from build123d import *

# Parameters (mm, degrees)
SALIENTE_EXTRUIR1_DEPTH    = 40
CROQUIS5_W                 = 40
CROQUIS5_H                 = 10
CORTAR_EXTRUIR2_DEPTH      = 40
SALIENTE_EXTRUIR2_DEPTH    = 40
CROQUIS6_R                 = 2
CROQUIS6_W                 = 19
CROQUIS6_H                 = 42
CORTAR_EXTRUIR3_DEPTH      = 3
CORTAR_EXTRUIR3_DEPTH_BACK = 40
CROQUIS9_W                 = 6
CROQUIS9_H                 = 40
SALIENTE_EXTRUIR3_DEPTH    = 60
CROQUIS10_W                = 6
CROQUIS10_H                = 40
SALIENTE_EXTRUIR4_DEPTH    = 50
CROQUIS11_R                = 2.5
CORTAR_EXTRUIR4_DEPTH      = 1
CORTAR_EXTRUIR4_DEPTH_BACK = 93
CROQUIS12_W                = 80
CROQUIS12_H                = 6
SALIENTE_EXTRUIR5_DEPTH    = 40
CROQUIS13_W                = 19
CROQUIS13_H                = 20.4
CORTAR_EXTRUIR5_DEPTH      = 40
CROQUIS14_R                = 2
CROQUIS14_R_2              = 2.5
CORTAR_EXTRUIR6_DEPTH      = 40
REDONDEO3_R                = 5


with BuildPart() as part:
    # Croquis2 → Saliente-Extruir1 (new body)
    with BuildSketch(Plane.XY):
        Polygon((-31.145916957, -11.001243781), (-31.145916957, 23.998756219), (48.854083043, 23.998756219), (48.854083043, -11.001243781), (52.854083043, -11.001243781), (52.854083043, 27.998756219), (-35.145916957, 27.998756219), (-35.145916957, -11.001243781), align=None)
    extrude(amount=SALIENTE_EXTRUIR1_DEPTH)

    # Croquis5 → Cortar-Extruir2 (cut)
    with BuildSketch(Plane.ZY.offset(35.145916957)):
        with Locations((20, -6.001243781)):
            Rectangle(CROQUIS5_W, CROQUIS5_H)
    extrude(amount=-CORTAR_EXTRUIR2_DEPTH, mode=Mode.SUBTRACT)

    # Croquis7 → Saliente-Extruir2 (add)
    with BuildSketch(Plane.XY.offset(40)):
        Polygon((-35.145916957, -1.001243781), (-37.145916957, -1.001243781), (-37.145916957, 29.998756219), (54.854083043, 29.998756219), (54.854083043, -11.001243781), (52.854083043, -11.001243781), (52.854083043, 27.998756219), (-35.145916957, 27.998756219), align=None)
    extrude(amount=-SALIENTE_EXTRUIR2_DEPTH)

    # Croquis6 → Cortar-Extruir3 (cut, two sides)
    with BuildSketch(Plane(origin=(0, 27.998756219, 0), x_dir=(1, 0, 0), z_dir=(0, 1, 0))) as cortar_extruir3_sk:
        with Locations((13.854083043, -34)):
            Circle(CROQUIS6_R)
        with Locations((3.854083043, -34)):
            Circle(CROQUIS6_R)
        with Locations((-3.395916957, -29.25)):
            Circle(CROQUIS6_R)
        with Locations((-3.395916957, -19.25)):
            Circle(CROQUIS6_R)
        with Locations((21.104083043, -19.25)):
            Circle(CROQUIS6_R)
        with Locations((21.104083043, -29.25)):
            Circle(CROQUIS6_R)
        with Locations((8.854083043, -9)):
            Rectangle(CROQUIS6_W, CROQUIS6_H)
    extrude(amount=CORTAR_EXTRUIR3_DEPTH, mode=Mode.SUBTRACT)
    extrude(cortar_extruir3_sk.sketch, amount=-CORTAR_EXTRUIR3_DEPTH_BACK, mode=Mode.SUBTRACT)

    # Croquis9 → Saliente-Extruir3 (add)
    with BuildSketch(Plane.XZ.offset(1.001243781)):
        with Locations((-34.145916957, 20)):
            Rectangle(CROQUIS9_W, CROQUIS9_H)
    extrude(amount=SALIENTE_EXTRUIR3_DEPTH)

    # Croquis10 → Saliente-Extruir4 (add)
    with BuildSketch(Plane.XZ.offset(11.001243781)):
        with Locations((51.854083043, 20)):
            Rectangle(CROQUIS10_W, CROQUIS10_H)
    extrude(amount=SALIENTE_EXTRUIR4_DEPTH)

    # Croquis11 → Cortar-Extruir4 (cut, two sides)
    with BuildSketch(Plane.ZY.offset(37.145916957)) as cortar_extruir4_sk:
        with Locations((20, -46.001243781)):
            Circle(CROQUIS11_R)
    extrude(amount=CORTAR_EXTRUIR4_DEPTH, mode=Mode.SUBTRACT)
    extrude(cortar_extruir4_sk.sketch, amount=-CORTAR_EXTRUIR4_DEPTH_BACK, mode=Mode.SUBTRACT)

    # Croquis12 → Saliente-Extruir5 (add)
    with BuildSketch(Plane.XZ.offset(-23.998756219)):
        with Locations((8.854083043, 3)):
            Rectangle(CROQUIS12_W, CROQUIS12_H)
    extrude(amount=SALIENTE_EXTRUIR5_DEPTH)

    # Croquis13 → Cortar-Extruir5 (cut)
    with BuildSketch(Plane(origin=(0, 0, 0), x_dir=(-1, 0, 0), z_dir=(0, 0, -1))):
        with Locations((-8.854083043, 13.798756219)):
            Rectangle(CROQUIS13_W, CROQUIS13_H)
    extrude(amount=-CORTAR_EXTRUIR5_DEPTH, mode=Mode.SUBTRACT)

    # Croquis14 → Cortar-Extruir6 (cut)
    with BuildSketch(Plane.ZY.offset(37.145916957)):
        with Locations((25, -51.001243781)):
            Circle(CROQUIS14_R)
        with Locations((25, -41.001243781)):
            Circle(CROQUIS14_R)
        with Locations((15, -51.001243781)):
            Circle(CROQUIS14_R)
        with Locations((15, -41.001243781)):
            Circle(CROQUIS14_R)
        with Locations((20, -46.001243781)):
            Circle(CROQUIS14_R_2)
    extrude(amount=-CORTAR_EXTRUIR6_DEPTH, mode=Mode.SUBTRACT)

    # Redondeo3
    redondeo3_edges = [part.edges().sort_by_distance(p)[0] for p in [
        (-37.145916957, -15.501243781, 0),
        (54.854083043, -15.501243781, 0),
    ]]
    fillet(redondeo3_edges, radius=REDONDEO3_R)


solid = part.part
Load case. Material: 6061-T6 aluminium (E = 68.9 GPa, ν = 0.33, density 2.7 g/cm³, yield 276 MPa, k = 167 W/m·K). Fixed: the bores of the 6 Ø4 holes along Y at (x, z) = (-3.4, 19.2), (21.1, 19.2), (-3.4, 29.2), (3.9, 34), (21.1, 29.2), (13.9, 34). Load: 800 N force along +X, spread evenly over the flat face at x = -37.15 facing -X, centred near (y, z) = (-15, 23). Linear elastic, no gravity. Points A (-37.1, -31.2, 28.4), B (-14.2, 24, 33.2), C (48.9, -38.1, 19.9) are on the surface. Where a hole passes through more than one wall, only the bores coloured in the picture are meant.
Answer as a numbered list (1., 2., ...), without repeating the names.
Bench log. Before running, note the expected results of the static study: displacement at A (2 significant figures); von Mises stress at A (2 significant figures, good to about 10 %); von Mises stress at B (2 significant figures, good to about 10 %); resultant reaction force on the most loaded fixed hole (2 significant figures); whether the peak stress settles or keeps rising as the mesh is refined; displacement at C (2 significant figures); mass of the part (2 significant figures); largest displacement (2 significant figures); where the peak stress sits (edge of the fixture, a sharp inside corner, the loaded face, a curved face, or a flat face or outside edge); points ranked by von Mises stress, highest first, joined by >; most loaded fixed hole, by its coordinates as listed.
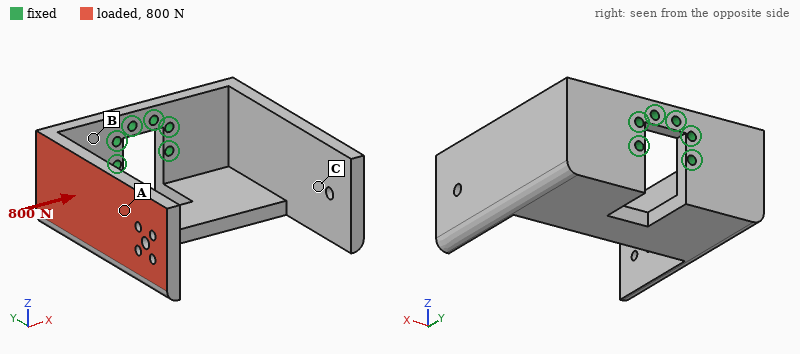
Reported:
1. 0.38 mm
2. 18 MPa
3. 38 MPa
4. 1.1 kN
5. keeps rising
6. 0.20 mm
7. 200 g
8. 0.71 mm
9. edge of the fixture
10. B > A > C
11. (21.1, 19.2)
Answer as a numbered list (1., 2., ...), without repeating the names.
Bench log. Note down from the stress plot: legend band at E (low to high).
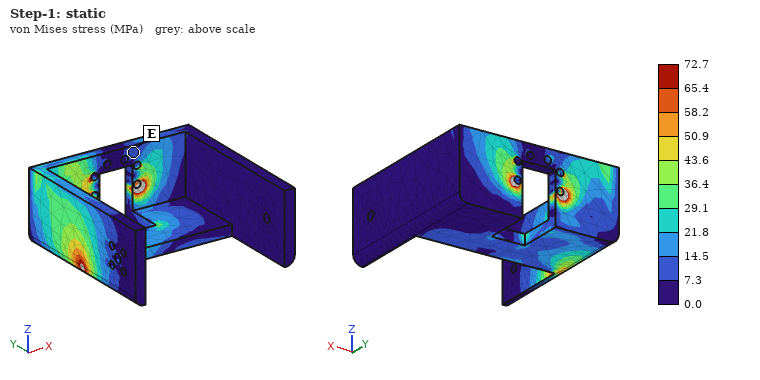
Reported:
1. 7.3 to 14.5 MPa
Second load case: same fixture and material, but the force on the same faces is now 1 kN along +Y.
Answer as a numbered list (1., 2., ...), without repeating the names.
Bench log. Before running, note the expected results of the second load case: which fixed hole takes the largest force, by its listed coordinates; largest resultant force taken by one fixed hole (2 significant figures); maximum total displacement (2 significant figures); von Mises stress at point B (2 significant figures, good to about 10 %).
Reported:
1. (-3.4, 19.2)
2. 1.3 kN
3. 0.30 mm
4. 40 MPa
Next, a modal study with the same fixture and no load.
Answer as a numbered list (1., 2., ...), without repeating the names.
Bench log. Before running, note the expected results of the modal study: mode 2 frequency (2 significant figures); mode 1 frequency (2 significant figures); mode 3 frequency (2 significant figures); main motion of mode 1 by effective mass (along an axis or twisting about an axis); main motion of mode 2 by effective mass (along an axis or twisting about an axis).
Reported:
1. 760 Hz
2. 690 Hz
3. 1200 Hz
4. along X
5. along Z
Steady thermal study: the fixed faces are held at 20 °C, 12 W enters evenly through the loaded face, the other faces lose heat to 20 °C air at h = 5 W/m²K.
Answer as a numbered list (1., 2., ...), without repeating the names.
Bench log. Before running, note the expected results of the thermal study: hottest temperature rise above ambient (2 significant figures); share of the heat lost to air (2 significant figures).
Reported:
1. 15 K
2. 4.8 %
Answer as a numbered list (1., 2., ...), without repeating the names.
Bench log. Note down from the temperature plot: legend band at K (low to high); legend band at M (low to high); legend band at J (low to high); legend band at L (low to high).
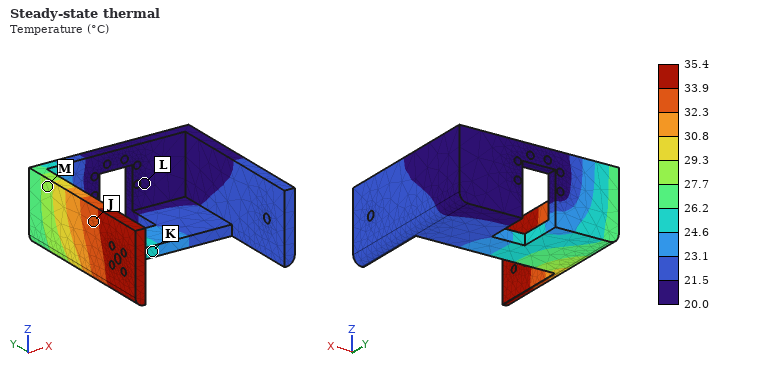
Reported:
1. 24.6 to 26.2 °C
2. 27.7 to 29.3 °C
3. 32.3 to 33.9 °C
4. 20.0 to 21.5 °C
